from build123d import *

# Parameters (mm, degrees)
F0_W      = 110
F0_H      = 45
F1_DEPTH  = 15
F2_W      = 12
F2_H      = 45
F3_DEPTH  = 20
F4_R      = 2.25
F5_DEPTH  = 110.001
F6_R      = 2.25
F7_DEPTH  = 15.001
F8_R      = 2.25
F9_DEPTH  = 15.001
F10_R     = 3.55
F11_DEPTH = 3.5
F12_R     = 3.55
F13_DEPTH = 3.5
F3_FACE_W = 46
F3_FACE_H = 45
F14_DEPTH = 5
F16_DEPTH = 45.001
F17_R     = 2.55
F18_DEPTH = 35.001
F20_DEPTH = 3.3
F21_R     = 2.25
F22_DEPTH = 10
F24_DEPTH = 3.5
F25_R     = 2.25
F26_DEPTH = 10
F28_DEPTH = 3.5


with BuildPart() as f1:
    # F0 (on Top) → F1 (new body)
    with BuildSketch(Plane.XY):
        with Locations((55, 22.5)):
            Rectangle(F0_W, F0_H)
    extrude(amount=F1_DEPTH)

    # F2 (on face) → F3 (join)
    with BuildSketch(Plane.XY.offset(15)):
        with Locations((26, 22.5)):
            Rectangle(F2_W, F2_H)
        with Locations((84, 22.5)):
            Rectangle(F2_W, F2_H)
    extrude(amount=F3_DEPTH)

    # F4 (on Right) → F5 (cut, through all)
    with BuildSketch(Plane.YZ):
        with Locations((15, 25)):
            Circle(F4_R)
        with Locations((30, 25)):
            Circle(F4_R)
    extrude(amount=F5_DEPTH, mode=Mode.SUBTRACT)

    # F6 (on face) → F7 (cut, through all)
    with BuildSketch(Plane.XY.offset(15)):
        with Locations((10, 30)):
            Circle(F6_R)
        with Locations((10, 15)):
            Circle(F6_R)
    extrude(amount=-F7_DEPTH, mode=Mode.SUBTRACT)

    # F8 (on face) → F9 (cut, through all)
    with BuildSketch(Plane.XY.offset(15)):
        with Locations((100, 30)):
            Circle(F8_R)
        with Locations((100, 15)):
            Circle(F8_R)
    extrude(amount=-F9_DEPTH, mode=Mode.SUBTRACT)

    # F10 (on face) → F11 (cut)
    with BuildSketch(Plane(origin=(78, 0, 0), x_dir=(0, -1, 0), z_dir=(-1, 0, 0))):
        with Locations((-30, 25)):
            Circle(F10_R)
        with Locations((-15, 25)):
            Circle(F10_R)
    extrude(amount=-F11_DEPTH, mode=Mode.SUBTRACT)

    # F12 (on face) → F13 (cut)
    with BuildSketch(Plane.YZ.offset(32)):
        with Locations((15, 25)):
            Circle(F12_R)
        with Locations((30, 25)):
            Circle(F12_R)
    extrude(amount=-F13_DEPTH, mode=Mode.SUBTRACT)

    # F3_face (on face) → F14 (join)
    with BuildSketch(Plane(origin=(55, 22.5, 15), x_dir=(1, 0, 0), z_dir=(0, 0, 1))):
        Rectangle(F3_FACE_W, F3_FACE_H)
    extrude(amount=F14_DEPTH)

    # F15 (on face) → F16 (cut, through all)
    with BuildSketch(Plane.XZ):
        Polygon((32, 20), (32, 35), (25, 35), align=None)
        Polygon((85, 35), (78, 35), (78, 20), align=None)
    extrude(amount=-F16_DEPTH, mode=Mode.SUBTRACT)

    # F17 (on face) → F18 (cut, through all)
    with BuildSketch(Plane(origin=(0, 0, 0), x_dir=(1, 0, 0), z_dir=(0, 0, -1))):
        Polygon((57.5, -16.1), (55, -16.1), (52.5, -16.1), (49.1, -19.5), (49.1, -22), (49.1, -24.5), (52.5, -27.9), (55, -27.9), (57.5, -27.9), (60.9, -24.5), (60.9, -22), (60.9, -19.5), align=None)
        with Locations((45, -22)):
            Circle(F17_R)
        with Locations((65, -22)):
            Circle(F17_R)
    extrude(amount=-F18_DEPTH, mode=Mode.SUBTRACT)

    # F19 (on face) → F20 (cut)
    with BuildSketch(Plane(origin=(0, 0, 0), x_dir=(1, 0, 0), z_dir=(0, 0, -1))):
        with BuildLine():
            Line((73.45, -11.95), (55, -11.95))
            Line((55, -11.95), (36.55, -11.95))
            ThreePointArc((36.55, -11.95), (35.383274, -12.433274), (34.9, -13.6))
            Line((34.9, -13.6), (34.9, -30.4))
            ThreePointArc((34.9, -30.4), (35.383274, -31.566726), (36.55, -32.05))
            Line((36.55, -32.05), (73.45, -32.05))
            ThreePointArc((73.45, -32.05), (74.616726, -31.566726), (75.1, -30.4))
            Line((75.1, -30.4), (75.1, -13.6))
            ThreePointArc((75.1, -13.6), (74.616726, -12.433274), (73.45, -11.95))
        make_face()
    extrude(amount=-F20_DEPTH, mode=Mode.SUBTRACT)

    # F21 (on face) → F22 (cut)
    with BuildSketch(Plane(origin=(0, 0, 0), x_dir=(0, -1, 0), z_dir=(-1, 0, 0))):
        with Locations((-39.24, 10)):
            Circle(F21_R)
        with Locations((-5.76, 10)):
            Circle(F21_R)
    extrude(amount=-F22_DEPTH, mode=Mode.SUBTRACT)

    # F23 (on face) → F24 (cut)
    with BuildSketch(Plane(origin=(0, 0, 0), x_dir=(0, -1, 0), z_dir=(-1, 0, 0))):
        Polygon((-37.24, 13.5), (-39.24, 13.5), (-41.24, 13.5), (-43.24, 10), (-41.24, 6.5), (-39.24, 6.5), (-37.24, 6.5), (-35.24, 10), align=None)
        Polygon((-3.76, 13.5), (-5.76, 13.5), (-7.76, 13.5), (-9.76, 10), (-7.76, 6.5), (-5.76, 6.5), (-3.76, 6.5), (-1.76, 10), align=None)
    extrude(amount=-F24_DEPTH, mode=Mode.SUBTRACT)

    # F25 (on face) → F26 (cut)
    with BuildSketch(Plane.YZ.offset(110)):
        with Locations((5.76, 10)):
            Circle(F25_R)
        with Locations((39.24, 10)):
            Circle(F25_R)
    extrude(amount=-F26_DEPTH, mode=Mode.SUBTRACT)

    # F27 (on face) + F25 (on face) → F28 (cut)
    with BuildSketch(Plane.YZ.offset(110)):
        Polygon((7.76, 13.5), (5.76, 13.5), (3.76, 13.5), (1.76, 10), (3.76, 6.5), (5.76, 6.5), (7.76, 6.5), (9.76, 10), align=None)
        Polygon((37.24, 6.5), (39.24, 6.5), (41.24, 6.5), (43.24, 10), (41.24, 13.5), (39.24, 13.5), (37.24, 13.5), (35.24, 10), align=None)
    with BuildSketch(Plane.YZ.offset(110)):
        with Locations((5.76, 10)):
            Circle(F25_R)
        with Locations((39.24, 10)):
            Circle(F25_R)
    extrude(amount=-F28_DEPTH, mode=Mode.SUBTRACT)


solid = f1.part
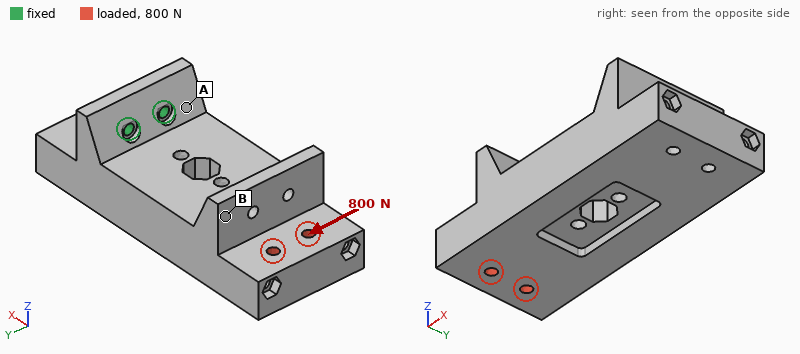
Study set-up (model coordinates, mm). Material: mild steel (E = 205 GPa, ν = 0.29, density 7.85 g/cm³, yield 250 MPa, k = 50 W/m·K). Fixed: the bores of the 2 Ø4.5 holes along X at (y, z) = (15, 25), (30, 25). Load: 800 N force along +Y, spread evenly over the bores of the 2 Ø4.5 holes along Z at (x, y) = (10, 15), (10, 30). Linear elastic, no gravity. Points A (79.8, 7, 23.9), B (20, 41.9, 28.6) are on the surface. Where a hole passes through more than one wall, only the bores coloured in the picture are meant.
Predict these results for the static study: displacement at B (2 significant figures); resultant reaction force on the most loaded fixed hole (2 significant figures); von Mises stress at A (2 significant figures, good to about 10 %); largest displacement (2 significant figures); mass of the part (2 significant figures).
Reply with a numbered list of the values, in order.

1. 24 µm
2. 2.7 kN
3. 13 MPa
4. 31 µm
5. 730 g
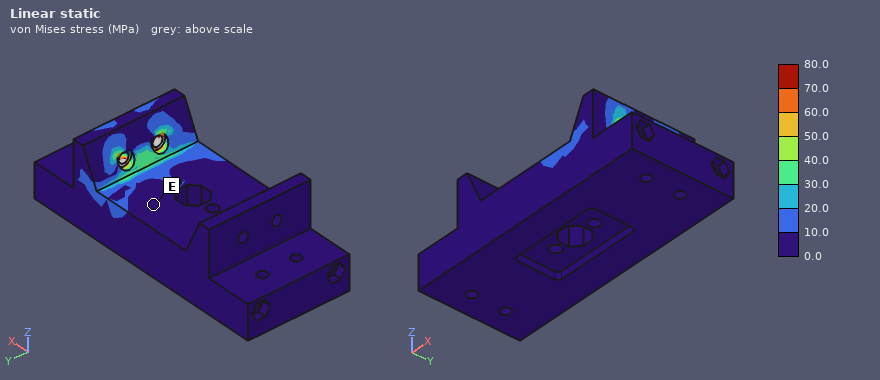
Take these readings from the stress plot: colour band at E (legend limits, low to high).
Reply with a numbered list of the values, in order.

1. 0.0 to 10.0 MPa
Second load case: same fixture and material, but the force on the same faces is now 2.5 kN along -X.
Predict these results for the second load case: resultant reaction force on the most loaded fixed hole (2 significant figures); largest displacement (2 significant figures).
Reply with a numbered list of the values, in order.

1. 1.3 kN
2. 60 µm
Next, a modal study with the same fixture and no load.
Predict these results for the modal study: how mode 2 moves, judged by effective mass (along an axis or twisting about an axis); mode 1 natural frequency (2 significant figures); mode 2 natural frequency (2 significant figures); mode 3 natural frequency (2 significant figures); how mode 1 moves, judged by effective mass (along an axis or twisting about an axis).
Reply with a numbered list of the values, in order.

1. along Y
2. 930 Hz
3. 1700 Hz
4. 4500 Hz
5. along Z
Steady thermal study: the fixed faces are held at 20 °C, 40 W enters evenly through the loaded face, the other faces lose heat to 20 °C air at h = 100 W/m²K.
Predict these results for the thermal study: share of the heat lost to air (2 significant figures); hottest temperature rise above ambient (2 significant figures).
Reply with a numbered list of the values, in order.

1. 79 %
2. 45 K
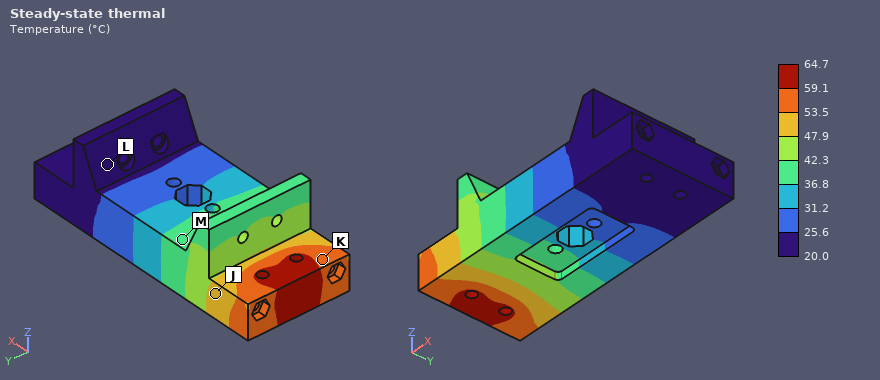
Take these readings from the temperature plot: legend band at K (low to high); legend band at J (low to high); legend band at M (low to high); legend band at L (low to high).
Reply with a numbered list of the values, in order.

1. 53.5 to 59.1 °C
2. 47.9 to 53.5 °C
3. 36.8 to 42.3 °C
4. 20.0 to 25.6 °C
